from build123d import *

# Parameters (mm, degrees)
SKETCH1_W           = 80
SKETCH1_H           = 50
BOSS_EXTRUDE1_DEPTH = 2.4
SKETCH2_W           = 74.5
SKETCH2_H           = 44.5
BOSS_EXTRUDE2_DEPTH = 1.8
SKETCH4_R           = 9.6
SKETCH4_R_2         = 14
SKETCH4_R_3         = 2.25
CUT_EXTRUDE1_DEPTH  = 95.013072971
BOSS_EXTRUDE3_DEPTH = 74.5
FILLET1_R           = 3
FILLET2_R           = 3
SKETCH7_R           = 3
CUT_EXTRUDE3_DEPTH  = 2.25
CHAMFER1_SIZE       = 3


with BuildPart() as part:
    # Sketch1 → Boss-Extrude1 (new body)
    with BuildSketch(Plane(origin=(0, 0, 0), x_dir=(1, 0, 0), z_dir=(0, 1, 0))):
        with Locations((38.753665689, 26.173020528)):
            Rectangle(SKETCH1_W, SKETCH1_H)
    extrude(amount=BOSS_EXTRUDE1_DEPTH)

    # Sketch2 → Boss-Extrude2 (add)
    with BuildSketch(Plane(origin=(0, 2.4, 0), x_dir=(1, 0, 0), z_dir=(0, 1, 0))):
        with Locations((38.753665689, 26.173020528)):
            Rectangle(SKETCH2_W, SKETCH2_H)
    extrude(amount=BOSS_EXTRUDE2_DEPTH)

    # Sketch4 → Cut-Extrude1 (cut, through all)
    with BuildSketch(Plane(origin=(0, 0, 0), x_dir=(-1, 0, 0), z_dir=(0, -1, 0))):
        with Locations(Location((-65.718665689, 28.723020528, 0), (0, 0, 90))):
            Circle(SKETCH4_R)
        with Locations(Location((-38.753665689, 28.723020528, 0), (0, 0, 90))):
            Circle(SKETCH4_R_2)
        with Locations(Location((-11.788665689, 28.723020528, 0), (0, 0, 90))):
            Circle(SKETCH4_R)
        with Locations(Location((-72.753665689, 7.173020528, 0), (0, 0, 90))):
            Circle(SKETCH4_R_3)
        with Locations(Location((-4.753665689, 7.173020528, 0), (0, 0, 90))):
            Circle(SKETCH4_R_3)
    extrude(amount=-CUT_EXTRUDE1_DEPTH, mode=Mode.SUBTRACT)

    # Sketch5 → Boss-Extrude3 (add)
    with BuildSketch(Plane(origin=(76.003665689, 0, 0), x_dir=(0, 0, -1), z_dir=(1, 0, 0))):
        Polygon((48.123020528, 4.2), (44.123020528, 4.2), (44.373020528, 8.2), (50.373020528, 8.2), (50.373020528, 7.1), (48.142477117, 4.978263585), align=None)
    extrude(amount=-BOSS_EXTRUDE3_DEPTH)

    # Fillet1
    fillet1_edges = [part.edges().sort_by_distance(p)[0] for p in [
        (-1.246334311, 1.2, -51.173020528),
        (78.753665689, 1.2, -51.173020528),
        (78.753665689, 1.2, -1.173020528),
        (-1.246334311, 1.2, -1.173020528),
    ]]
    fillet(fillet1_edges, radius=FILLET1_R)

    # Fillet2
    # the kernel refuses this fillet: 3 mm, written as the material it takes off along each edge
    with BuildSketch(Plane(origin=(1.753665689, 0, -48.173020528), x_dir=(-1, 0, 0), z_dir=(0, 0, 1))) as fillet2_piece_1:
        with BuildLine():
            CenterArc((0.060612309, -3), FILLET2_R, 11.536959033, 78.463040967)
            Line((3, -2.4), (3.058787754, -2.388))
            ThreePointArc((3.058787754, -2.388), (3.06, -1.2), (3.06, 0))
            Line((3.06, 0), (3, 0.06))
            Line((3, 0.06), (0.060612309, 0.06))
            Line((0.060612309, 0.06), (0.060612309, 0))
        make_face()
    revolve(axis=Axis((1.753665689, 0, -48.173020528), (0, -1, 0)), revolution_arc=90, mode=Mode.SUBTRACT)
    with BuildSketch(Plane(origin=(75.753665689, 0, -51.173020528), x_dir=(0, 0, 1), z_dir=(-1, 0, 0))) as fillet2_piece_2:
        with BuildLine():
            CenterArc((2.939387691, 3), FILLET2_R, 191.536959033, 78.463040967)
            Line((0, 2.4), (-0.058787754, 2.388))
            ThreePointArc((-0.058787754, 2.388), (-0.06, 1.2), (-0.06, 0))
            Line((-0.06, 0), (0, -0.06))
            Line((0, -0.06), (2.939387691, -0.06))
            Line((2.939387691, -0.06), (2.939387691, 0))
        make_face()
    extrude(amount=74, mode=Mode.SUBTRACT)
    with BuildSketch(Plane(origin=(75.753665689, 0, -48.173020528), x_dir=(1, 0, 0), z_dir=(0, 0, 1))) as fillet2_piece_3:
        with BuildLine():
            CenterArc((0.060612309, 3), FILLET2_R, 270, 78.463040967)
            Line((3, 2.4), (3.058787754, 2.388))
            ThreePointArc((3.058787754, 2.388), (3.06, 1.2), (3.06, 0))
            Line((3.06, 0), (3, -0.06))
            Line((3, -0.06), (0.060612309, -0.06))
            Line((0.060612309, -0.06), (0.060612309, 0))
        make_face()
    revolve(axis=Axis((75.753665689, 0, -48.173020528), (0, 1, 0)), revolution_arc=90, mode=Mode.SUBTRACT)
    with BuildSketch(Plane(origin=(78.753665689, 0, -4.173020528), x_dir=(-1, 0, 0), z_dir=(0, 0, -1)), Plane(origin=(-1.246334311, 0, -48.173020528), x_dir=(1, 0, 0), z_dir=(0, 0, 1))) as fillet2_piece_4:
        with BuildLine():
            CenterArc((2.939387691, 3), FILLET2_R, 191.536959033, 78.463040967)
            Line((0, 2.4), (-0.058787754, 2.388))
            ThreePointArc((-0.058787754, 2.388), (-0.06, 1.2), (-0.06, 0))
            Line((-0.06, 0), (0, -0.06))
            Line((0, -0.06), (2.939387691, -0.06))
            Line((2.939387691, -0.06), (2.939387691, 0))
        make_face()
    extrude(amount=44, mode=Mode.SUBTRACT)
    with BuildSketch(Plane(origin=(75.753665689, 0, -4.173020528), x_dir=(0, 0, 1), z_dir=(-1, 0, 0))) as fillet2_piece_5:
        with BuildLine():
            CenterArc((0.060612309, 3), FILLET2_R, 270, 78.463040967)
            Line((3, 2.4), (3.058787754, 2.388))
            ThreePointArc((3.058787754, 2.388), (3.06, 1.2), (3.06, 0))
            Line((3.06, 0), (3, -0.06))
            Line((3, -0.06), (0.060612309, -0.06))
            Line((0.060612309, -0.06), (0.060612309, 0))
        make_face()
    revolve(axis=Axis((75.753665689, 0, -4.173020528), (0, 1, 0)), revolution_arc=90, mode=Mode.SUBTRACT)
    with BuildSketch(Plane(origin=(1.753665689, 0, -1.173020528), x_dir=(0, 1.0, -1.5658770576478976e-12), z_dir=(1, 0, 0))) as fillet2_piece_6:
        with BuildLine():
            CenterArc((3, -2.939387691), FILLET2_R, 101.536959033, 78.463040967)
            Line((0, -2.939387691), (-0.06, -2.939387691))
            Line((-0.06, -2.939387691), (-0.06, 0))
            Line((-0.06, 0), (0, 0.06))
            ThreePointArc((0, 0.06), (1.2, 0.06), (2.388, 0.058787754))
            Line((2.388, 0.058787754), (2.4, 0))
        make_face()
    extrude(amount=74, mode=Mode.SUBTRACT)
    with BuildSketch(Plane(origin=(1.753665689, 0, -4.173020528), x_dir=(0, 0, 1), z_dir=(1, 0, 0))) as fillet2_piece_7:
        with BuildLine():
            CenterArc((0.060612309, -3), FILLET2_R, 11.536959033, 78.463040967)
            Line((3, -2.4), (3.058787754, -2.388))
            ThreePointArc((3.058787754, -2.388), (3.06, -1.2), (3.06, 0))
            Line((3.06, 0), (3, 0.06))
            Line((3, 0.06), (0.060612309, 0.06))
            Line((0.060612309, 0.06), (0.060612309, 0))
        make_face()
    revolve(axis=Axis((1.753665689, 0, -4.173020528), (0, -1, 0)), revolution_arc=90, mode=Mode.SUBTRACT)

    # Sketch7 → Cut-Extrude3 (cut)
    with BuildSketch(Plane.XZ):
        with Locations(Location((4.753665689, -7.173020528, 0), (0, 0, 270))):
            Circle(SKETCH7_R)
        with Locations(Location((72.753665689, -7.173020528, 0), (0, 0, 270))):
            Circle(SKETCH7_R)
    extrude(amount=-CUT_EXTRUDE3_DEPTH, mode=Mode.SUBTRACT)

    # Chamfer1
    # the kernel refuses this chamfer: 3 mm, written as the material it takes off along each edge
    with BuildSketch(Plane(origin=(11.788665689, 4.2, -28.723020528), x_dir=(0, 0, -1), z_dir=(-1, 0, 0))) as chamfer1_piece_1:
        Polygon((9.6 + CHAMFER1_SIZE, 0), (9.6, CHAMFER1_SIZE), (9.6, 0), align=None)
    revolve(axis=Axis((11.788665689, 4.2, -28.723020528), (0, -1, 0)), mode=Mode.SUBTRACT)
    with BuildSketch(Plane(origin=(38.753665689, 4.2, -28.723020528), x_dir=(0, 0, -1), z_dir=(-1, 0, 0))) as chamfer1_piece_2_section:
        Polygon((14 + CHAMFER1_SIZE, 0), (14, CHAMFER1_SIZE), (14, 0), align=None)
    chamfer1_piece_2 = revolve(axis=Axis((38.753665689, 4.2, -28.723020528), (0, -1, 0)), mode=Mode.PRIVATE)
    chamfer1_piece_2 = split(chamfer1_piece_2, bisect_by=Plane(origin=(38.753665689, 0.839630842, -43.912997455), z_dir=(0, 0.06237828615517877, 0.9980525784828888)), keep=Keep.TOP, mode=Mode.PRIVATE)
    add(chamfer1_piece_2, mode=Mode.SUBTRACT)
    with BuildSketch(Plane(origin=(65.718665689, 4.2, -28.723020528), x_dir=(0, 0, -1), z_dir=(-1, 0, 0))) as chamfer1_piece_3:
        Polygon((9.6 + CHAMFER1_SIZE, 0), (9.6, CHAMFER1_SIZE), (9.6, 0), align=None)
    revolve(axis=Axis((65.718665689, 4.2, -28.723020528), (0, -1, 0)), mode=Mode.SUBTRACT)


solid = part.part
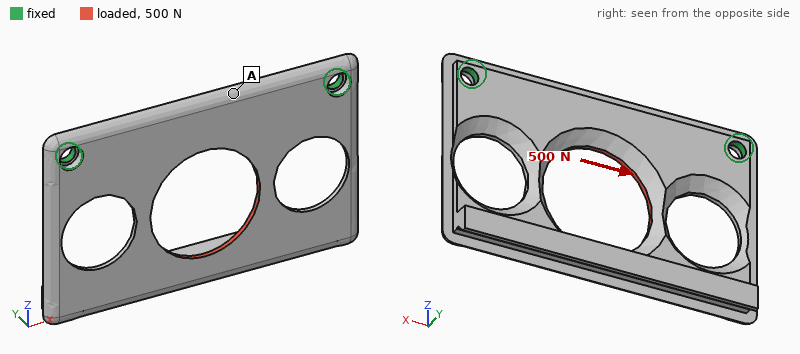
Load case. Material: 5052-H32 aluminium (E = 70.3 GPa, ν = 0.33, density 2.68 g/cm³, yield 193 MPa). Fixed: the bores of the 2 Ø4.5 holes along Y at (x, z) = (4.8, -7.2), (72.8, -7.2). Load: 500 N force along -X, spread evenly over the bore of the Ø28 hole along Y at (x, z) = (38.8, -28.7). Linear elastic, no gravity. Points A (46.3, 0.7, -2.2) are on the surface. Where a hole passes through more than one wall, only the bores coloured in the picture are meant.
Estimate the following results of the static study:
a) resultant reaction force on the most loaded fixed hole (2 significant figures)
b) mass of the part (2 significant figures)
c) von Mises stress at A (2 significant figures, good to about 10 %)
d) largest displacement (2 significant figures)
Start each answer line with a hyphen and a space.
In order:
- 290 N
- 28 g
- 5.1 MPa
- 29 µm
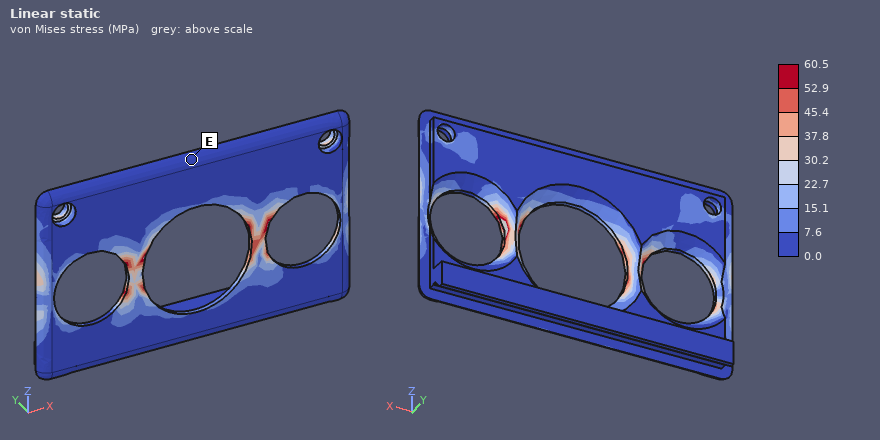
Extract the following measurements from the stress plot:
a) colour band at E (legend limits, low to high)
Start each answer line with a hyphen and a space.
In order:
- 0.0 to 7.6 MPa
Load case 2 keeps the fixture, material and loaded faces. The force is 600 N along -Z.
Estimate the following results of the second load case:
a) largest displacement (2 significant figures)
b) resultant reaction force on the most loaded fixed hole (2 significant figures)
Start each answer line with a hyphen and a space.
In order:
- 0.12 mm
- 320 N
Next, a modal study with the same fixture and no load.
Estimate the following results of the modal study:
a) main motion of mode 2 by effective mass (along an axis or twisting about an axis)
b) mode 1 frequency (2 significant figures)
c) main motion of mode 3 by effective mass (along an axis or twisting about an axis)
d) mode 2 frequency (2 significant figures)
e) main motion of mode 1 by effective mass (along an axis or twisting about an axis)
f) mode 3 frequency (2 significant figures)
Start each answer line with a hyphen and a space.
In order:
- twisting about Z
- 610 Hz
- along Y
- 1700 Hz
- along Y
- 3800 Hz
